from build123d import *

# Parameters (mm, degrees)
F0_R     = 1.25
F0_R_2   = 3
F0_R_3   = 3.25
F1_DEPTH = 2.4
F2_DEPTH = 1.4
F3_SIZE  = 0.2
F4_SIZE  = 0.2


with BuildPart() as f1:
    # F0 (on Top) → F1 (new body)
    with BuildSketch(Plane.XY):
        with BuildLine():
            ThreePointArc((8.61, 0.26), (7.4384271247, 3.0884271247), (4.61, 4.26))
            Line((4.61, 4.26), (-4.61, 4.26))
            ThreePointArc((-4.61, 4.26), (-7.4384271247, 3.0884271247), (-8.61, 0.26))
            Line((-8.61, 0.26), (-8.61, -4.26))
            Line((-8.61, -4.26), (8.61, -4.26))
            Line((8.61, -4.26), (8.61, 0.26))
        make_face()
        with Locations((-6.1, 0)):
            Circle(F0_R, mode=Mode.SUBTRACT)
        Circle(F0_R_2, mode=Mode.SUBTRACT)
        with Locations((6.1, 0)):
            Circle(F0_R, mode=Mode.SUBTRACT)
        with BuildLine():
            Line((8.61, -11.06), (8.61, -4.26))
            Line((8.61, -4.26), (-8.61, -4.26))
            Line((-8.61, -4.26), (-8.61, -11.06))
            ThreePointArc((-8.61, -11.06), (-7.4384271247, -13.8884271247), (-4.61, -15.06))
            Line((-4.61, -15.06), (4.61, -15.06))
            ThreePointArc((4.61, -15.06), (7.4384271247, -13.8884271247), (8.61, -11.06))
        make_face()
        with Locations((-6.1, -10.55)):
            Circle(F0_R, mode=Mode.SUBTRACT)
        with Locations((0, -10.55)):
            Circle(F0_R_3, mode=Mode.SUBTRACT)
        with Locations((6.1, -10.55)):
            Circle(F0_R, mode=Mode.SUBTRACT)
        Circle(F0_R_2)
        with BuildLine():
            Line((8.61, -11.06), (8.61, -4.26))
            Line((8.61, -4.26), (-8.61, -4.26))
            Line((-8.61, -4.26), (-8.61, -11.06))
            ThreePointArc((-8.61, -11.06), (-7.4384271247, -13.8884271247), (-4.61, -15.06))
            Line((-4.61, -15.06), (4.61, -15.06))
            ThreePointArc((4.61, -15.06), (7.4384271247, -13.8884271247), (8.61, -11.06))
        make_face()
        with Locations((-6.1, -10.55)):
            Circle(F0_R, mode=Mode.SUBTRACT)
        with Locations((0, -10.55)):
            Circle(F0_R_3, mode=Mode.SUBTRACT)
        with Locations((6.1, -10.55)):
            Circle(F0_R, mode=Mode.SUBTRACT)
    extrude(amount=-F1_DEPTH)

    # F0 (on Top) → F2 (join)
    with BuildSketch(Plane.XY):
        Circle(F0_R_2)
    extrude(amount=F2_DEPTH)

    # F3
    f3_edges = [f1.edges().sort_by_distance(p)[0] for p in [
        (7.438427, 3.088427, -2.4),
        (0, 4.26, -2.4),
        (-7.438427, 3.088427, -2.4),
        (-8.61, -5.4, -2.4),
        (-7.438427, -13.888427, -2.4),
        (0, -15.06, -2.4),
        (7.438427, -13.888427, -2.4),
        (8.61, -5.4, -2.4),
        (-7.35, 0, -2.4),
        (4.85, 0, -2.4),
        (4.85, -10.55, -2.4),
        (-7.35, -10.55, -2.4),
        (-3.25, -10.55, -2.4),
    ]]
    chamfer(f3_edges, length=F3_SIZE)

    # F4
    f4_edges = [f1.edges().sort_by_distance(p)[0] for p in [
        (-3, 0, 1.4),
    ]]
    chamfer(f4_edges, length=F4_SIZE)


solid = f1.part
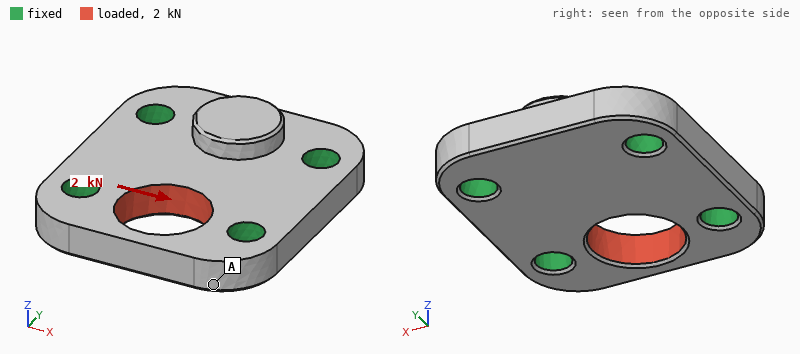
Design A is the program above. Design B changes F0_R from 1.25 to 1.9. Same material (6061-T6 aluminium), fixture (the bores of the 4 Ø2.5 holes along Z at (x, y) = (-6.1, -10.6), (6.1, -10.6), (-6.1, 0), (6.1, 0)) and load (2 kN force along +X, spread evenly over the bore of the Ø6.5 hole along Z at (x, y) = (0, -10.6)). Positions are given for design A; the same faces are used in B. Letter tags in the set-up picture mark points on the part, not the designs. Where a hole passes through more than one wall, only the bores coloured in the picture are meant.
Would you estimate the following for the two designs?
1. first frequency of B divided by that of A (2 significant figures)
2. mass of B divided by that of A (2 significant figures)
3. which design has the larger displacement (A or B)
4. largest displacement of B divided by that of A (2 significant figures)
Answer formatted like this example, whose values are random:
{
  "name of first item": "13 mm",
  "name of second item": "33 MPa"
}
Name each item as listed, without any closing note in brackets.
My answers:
{
  "first frequency of B divided by that of A": "1.2",
  "mass of B divided by that of A": "0.91",
  "which design has the larger displacement": "A",
  "largest displacement of B divided by that of A": "0.76"
}
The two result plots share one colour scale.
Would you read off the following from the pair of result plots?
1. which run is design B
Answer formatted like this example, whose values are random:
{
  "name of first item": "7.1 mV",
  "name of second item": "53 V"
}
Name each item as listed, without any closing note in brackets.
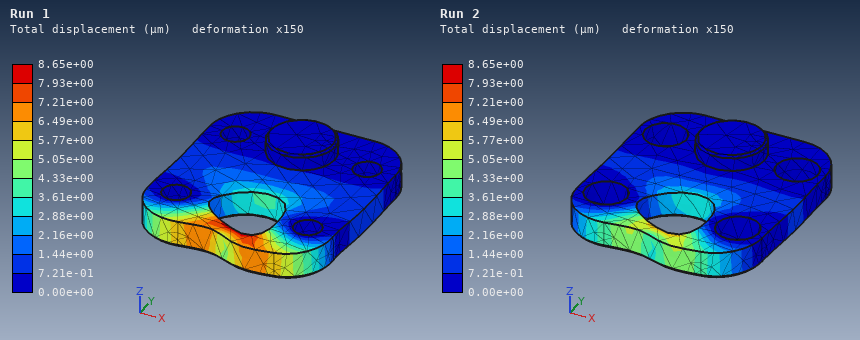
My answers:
{
  "which run is design B": "Run 2"
}
